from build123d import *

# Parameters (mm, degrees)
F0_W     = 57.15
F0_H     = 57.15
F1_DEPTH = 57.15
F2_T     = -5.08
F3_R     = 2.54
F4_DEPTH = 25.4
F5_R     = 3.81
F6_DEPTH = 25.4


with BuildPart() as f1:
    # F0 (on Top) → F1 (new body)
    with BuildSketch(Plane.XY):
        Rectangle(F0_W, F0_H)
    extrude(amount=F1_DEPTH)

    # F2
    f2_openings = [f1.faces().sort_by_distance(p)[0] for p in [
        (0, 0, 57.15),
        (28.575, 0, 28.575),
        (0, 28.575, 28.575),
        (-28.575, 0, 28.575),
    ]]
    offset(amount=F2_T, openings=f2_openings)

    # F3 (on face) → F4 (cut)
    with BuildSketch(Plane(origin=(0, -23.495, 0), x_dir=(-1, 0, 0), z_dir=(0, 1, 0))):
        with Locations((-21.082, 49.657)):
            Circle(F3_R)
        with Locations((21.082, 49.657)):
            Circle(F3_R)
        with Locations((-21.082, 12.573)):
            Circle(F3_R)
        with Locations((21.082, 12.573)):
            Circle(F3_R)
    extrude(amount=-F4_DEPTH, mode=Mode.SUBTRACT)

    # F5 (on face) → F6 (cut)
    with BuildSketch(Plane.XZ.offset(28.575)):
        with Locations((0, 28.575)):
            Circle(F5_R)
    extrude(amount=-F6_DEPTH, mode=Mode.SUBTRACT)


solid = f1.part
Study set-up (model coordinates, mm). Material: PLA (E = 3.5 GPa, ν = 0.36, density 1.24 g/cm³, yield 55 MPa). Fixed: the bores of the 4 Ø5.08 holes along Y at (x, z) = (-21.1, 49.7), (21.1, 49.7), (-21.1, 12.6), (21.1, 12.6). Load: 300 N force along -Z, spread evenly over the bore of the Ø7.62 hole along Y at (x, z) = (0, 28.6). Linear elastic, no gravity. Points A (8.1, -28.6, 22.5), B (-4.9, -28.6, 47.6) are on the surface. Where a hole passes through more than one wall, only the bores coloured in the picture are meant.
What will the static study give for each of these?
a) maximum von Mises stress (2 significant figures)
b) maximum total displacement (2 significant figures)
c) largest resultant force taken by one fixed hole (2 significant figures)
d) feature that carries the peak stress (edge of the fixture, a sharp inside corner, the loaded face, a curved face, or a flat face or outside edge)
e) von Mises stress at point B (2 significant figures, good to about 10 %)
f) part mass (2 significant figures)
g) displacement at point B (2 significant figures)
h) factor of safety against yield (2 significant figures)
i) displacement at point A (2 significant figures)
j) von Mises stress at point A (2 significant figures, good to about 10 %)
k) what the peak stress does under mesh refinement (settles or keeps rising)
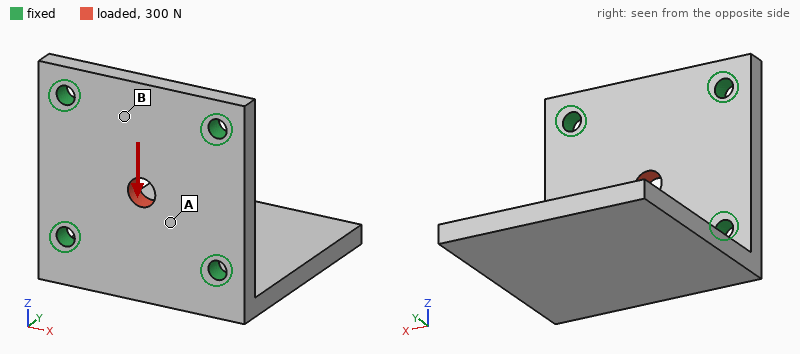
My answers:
4.3 MPa
13 µm
86 N
the loaded face
0.57 MPa
39 g
6.9 µm
13
7.2 µm
1.3 MPa
settles
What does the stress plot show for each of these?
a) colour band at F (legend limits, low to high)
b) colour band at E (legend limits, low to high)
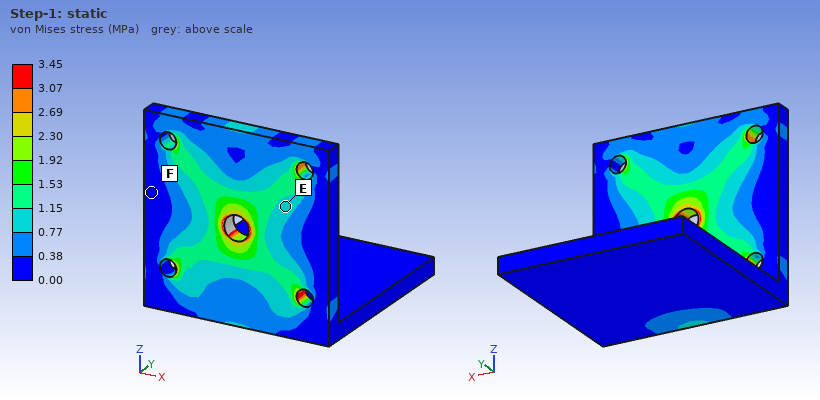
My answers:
0.00 to 0.38 MPa
0.77 to 1.15 MPa
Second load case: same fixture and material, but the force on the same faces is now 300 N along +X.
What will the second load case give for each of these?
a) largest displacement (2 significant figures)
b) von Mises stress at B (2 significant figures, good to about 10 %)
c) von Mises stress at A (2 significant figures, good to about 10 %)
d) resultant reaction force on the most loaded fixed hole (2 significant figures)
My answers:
12 µm
0.41 MPa
1.5 MPa
91 N
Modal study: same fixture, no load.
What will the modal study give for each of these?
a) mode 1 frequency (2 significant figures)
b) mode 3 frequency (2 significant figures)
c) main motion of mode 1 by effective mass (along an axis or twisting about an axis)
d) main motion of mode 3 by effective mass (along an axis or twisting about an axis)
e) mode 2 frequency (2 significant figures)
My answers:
370 Hz
1600 Hz
along Z
along X
950 Hz
